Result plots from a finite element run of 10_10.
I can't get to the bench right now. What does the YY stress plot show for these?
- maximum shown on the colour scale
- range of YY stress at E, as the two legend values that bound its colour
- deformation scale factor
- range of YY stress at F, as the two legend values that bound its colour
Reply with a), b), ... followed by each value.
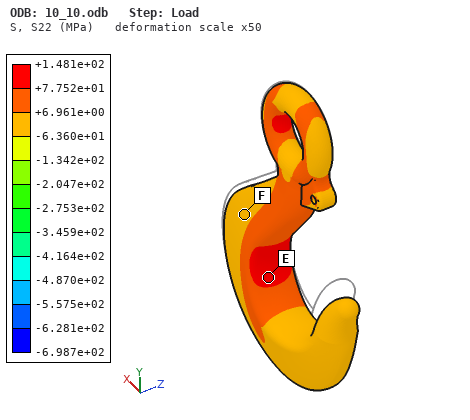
a) +1.481e+02 MPa
b) +7.752e+01 to +1.481e+02 MPa
c) 50
d) -6.360e+01 to +6.961e+00 MPa
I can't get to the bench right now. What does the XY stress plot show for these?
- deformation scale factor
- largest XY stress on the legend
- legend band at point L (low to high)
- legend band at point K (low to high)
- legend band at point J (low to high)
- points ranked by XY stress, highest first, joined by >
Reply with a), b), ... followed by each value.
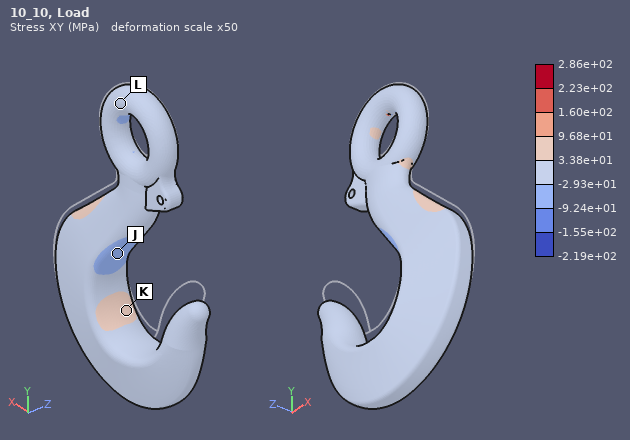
a) 50
b) 2.86e+02 MPa
c) -2.93e+01 to 3.38e+01 MPa
d) 3.38e+01 to 9.68e+01 MPa
e) -9.24e+01 to -2.93e+01 MPa
f) K > L > J
